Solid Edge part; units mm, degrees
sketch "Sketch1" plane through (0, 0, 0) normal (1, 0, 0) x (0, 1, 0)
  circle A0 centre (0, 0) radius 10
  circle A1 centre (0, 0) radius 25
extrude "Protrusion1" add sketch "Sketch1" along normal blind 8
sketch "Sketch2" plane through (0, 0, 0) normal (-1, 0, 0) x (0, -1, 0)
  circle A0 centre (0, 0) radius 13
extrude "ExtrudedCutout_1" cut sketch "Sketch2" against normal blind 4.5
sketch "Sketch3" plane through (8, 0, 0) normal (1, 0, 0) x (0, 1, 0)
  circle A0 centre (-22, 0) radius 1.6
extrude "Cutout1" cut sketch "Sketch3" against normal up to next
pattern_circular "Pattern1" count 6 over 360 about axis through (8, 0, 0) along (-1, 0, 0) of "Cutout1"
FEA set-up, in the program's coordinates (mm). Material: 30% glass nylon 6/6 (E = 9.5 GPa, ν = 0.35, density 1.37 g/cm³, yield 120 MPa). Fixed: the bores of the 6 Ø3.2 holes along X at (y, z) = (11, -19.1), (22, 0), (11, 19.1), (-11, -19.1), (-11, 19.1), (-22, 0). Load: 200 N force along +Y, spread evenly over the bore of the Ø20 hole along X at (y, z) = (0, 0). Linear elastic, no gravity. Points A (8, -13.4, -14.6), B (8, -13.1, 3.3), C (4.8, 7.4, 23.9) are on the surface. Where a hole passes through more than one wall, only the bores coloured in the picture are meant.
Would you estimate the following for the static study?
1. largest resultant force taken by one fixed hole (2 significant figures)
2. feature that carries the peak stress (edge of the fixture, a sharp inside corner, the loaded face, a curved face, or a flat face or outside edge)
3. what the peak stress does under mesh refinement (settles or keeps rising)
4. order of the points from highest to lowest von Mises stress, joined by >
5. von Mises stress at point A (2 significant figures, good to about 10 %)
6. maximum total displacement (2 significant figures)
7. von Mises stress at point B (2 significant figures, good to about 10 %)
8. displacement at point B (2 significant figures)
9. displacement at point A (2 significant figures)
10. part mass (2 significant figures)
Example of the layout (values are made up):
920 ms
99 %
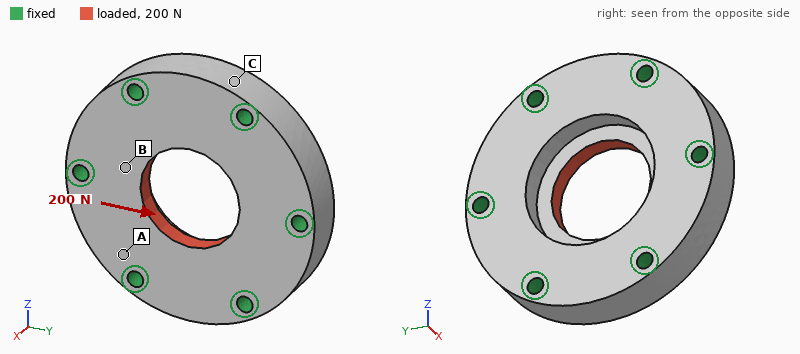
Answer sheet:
47 N
edge of the fixture
keeps rising
B > A > C
0.44 MPa
1.7 µm
1.0 MPa
1.2 µm
0.48 µm
16 g
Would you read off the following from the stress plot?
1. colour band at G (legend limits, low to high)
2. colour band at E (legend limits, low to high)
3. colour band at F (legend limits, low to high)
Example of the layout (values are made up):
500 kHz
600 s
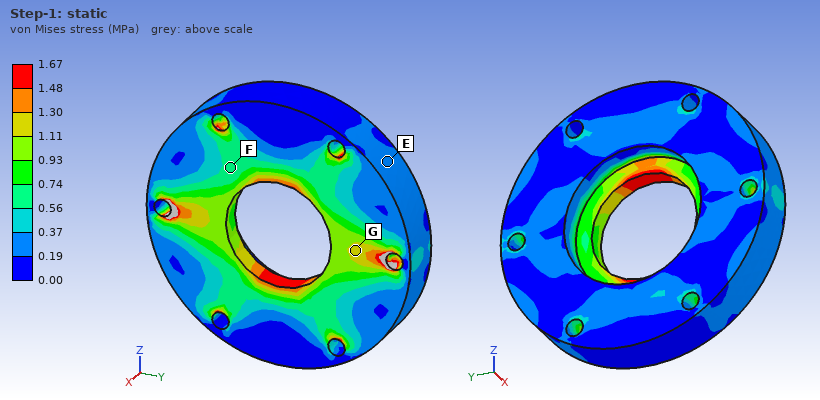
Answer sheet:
1.11 to 1.30 MPa
0.19 to 0.37 MPa
0.56 to 0.74 MPa
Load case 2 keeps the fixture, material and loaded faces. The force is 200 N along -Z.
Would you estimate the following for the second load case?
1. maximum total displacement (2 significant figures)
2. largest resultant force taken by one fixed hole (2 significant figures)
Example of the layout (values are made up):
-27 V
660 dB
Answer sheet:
1.8 µm
42 N
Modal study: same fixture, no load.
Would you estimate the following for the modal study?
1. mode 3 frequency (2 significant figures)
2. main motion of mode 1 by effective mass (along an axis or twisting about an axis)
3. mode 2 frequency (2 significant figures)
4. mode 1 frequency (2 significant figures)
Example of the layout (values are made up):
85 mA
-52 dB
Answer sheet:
23 kHz
along X
23 kHz
20 kHz
